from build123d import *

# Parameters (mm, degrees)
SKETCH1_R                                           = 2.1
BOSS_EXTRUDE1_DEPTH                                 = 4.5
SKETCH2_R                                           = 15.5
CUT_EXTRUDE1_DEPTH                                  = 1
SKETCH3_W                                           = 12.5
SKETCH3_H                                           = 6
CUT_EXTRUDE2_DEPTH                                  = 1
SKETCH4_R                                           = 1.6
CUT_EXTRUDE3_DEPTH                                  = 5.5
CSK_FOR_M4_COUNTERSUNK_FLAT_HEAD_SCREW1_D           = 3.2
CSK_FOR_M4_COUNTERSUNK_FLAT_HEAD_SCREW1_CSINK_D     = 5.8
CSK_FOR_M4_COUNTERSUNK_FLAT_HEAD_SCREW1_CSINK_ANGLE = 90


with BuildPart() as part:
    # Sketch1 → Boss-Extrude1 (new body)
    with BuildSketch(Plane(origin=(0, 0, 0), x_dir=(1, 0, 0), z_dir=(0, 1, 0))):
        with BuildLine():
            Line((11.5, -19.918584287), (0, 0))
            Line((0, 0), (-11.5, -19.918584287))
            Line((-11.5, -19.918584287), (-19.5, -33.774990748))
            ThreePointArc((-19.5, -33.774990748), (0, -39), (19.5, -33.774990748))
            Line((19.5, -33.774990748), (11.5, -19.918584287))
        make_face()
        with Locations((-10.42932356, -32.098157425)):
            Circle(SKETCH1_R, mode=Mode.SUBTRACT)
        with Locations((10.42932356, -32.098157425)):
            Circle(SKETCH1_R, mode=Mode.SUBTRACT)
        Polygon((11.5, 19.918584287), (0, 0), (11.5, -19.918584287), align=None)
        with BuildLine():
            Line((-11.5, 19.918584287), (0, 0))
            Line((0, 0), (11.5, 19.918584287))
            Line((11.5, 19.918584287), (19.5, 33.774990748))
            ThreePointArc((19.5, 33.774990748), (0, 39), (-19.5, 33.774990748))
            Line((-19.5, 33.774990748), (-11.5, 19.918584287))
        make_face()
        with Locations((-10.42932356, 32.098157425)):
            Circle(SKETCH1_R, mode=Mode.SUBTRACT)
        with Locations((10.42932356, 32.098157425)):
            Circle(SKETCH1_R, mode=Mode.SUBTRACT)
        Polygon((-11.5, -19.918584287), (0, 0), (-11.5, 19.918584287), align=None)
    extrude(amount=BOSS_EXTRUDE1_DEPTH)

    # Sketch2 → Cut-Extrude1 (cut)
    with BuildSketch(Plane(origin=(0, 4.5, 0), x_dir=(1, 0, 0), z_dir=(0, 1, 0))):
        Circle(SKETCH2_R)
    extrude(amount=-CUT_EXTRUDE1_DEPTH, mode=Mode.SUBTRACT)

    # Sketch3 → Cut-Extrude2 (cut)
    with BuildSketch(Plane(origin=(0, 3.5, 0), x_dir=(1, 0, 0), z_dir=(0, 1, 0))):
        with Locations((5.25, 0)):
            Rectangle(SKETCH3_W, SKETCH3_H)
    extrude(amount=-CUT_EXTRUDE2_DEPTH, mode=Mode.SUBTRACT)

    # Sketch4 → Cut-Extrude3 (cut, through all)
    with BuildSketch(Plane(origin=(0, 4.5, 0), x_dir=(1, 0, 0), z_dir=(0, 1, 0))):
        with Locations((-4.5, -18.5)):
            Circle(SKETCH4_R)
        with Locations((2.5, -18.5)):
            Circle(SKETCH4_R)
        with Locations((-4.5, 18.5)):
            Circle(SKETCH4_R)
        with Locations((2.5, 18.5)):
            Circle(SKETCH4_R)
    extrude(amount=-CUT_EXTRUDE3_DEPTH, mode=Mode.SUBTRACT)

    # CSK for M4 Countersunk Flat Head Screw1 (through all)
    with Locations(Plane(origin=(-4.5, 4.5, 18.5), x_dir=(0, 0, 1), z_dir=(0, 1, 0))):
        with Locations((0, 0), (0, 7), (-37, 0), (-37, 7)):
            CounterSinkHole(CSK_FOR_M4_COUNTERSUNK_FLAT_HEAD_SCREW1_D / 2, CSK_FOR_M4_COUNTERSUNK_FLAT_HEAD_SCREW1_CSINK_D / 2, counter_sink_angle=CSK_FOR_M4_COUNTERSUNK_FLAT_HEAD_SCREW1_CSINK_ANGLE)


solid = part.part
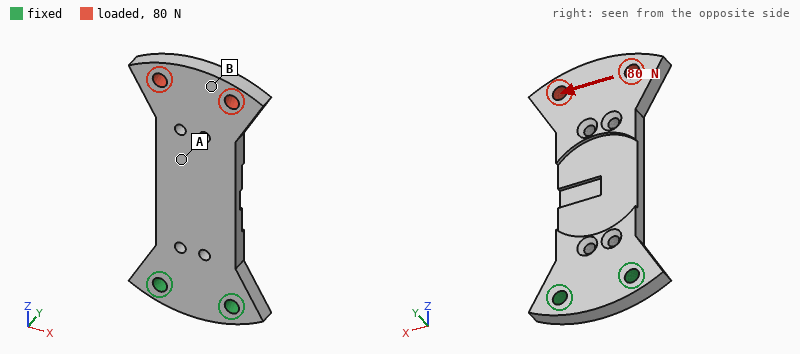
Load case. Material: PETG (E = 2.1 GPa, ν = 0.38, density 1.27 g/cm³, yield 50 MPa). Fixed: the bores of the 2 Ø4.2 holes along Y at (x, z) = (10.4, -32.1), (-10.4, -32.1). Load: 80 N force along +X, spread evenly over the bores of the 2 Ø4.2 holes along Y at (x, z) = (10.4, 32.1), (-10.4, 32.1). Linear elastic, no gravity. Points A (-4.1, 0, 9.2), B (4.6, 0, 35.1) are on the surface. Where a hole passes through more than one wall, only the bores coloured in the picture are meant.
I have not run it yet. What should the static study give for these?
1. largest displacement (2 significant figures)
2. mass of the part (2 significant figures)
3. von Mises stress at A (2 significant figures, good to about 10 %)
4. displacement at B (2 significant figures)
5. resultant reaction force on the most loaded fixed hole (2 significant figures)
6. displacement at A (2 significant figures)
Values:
1.0 mm
10 g
3.2 MPa
0.86 mm
230 N
0.37 mm
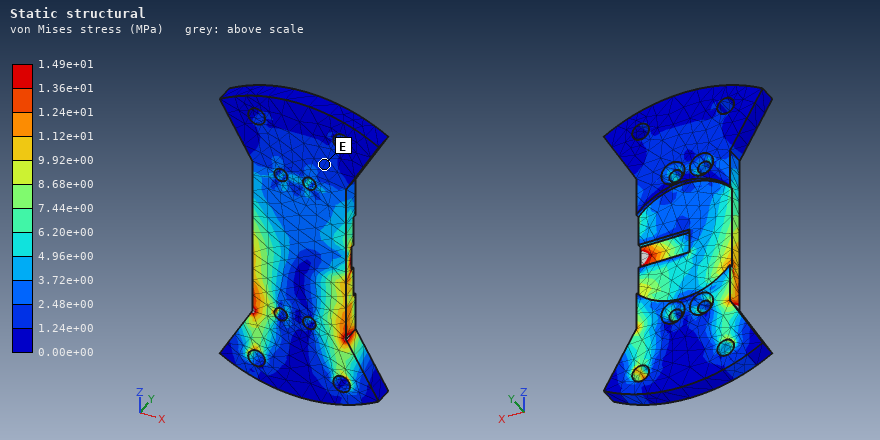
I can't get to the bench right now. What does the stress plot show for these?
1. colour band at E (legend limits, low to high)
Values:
1.24e+00 to 2.48e+00 MPa
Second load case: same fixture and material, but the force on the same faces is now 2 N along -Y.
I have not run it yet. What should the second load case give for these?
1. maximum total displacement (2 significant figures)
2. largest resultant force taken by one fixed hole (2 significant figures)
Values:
0.84 mm
1.1 N
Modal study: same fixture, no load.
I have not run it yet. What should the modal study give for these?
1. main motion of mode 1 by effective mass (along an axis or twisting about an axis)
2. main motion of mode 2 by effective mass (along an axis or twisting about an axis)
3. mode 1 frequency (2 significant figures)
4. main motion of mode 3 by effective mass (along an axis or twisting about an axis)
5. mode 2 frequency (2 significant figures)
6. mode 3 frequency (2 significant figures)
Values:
along Y
twisting about Z
150 Hz
along X
650 Hz
860 Hz
